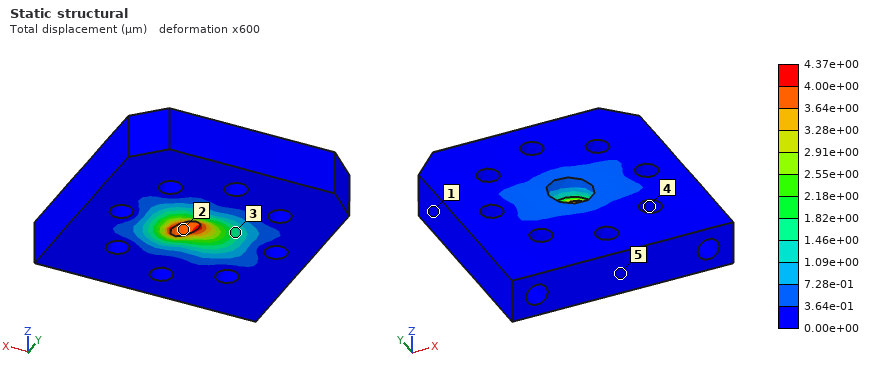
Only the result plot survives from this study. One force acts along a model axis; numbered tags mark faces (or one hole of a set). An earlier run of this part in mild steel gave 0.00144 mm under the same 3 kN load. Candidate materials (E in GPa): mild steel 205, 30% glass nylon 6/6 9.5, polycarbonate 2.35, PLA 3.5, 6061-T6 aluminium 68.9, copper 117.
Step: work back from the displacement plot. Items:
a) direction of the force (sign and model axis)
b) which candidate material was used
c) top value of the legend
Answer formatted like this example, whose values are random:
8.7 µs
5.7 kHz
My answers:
+X
6061-T6 aluminium
4.37e+00 µm
